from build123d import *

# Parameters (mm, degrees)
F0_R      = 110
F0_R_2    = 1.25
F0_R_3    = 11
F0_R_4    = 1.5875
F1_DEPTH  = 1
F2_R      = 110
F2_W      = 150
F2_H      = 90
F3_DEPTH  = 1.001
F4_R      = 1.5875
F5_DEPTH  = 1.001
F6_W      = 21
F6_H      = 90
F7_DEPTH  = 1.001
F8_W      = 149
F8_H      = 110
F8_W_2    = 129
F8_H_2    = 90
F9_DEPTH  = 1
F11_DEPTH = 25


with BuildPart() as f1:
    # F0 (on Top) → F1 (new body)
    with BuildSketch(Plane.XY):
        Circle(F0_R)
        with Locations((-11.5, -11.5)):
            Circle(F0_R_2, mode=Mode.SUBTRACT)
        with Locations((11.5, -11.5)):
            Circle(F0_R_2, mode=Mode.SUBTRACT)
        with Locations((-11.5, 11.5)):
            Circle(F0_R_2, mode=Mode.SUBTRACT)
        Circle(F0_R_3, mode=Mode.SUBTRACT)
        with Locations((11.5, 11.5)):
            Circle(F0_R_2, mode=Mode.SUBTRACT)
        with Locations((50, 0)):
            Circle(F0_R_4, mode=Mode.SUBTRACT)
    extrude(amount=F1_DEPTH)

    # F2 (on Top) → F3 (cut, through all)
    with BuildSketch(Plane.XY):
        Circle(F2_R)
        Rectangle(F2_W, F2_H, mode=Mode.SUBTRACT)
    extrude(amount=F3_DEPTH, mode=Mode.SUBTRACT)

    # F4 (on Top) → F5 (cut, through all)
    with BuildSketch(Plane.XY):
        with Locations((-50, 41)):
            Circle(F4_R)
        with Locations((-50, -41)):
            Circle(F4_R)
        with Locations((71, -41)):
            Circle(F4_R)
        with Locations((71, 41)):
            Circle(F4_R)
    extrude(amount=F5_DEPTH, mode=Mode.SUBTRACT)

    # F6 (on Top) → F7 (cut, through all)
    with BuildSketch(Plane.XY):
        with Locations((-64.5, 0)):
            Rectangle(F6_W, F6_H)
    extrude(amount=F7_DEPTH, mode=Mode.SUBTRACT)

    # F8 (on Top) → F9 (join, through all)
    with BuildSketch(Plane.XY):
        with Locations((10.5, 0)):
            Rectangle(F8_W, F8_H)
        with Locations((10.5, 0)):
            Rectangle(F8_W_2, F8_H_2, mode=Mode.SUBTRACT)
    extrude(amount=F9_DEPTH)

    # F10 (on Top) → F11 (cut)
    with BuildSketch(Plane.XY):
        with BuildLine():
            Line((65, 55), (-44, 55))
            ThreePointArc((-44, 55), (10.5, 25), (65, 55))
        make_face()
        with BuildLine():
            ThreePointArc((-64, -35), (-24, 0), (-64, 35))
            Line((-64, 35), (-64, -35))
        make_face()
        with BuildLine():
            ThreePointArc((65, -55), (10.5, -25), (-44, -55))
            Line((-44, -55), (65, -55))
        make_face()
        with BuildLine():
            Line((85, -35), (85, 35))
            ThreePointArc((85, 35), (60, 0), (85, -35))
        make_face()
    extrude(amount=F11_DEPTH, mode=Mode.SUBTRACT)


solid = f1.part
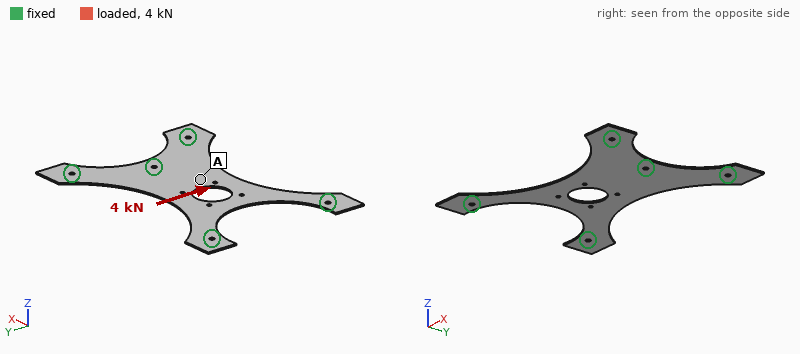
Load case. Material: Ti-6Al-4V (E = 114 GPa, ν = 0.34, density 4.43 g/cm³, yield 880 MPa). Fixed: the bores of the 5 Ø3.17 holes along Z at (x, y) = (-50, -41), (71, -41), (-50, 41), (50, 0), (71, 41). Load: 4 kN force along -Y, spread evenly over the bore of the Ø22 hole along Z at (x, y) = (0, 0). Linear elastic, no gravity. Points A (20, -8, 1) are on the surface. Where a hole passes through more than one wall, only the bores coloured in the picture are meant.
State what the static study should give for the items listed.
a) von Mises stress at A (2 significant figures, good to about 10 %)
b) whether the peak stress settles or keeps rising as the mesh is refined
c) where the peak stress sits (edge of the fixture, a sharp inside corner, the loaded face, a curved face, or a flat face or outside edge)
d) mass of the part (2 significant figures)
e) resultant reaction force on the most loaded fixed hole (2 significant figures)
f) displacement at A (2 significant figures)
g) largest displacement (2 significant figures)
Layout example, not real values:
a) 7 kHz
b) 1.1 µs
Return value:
a) 80 MPa
b) keeps rising
c) edge of the fixture
d) 34 g
e) 1.4 kN
f) 0.059 mm
g) 0.12 mm
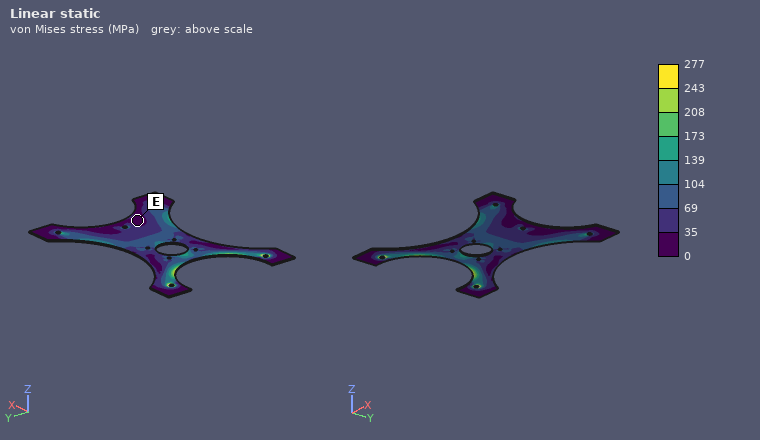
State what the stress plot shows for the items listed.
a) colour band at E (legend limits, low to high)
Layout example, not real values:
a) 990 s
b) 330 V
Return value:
a) 0 to 35 MPa
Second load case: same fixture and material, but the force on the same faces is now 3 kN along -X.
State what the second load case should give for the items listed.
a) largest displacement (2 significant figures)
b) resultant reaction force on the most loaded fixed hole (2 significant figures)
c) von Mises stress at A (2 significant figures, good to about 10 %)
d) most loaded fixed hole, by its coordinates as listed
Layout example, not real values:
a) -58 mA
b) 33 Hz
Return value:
a) 39 µm
b) 1.2 kN
c) 46 MPa
d) (50, 0)
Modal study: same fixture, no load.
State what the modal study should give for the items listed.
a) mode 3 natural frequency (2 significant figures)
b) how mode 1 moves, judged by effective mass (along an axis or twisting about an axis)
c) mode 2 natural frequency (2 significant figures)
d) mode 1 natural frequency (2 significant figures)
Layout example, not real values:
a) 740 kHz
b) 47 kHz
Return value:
a) 1000 Hz
b) along Z
c) 730 Hz
d) 430 Hz
